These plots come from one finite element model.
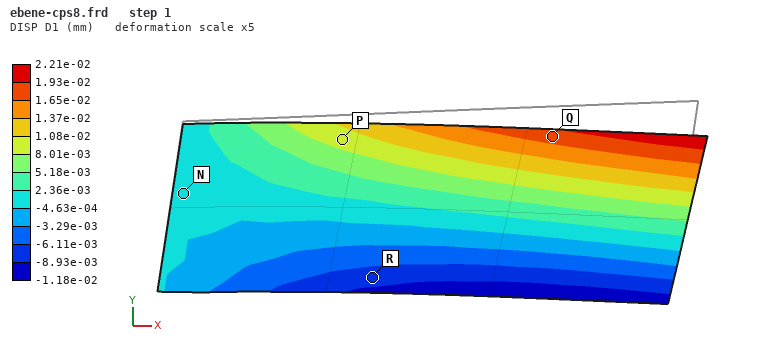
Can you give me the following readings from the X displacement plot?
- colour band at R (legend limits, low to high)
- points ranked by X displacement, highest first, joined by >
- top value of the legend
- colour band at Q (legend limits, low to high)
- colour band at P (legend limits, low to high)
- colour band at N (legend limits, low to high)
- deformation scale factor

-8.93e-03 to -6.11e-03 mm
Q > P > N > R
2.21e-02 mm
1.65e-02 to 1.93e-02 mm
8.01e-03 to 1.08e-02 mm
-4.63e-04 to 2.36e-03 mm
5
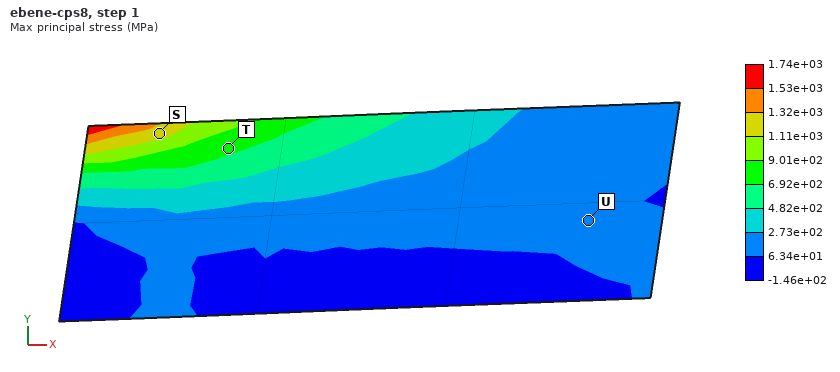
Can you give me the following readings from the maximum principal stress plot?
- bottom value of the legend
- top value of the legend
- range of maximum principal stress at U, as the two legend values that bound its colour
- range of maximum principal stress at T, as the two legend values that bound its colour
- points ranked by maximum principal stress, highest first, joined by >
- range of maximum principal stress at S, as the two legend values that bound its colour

-1.46e+02 MPa
1.74e+03 MPa
6.34e+01 to 2.73e+02 MPa
6.92e+02 to 9.01e+02 MPa
S > T > U
1.11e+03 to 1.32e+03 MPa
